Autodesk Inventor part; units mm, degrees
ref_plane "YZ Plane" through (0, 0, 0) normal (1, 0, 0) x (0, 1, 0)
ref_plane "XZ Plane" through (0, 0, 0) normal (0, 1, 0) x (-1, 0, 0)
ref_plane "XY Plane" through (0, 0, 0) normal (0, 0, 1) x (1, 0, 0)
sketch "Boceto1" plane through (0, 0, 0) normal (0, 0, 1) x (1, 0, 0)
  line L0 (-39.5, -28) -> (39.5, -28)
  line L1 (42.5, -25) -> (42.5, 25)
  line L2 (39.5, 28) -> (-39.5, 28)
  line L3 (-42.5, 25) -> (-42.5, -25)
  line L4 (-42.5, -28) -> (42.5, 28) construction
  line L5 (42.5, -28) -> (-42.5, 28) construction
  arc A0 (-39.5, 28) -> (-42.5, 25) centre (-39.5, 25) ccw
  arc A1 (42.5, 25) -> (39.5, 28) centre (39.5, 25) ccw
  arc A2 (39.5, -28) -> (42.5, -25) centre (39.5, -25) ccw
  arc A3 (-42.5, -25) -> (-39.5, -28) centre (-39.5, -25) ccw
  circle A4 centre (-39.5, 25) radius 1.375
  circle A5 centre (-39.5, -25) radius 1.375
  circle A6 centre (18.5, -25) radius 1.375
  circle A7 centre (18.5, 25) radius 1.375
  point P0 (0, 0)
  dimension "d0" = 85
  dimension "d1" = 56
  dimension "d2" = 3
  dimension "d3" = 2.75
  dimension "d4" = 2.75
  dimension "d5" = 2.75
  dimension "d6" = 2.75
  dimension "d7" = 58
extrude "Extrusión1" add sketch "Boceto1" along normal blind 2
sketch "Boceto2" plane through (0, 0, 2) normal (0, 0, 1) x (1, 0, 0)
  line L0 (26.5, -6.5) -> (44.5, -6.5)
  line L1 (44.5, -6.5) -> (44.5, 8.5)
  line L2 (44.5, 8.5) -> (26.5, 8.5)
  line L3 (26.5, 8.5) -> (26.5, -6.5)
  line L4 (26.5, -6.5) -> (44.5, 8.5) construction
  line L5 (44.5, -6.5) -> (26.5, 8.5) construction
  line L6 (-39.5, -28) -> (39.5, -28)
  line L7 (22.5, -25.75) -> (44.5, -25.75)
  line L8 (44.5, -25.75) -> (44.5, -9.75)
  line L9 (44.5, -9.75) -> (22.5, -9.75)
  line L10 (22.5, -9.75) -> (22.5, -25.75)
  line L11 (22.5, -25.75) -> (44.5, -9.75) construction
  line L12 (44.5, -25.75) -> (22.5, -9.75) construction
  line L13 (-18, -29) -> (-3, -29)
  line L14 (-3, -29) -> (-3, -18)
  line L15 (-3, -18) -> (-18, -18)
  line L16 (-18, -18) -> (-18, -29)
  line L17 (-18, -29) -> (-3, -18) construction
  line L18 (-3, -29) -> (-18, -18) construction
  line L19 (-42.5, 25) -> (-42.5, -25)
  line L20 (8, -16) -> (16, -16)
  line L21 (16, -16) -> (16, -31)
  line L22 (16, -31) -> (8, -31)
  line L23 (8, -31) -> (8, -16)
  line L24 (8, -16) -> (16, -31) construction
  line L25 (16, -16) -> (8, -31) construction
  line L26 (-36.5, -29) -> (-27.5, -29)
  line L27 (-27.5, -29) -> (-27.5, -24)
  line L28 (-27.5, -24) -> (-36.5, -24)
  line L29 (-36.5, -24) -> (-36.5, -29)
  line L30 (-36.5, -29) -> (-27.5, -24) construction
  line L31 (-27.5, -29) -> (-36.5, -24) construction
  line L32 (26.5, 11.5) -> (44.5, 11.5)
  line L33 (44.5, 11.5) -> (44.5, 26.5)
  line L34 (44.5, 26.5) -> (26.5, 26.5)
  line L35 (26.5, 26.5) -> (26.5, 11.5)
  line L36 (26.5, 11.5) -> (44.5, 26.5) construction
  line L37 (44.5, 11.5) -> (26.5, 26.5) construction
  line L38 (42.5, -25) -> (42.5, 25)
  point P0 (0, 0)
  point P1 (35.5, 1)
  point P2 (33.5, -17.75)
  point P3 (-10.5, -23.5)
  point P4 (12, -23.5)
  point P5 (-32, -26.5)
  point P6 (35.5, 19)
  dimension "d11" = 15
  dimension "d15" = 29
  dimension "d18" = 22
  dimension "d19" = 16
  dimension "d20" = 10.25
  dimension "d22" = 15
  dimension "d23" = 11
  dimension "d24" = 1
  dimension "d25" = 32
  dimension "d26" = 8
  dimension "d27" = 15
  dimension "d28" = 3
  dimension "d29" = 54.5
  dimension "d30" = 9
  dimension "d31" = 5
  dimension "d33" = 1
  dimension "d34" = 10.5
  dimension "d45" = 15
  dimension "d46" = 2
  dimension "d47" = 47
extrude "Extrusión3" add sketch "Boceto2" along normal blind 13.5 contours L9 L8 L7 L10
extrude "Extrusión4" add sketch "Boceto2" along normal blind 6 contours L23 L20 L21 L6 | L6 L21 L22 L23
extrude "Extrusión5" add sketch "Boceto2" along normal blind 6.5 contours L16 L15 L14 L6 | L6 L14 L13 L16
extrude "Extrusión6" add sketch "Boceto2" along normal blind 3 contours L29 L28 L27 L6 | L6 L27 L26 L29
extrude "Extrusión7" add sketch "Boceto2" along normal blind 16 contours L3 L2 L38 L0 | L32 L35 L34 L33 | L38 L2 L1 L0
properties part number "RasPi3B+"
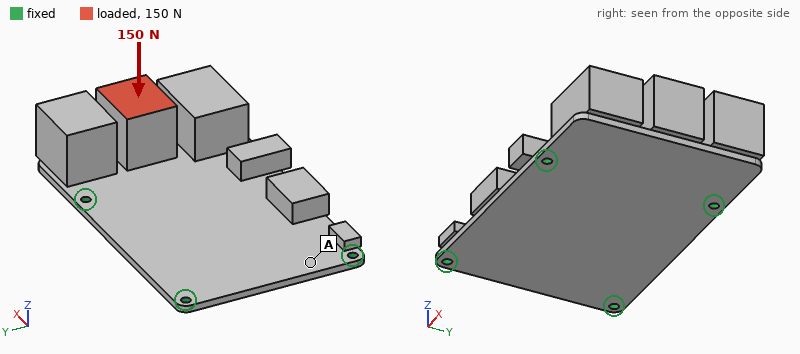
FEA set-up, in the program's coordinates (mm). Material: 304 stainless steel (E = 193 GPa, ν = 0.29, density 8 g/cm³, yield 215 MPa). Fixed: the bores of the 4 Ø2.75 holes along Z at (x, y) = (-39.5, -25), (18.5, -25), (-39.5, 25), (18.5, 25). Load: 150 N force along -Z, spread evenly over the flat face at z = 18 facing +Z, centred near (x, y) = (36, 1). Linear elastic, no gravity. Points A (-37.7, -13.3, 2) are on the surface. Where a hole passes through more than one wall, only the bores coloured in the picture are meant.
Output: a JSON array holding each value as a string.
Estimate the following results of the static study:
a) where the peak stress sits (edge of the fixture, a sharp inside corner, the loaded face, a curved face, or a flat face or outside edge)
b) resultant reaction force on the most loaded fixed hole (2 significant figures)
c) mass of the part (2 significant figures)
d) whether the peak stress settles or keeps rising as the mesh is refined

["edge of the fixture", "84 N", "200 g", "keeps rising"]
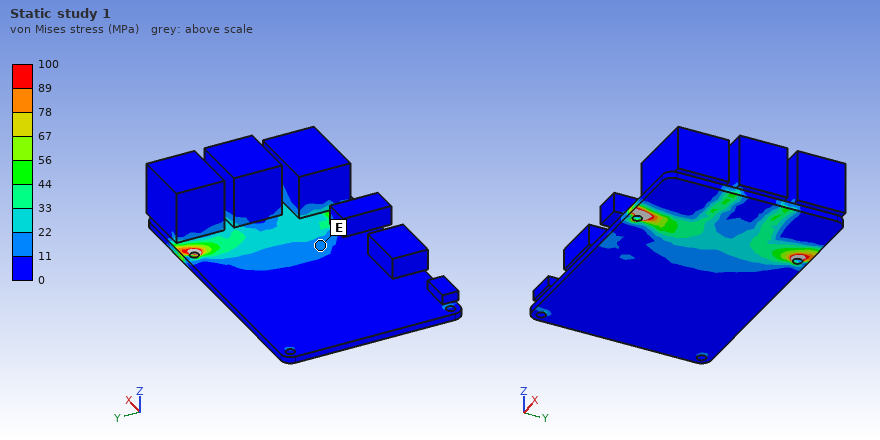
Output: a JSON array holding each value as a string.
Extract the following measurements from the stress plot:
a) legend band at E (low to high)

["11 to 22 MPa"]
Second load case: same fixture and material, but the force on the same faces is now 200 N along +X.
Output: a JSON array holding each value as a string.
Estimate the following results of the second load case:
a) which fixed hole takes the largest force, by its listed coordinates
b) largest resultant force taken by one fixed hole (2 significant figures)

["(18.5, 25)", "83 N"]
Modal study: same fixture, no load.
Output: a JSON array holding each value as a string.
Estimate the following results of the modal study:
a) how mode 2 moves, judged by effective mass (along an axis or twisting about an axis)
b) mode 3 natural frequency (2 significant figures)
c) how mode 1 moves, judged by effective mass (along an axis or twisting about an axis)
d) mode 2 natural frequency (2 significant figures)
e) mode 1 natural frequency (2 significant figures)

["along Z", "2400 Hz", "along Z", "2100 Hz", "690 Hz"]
